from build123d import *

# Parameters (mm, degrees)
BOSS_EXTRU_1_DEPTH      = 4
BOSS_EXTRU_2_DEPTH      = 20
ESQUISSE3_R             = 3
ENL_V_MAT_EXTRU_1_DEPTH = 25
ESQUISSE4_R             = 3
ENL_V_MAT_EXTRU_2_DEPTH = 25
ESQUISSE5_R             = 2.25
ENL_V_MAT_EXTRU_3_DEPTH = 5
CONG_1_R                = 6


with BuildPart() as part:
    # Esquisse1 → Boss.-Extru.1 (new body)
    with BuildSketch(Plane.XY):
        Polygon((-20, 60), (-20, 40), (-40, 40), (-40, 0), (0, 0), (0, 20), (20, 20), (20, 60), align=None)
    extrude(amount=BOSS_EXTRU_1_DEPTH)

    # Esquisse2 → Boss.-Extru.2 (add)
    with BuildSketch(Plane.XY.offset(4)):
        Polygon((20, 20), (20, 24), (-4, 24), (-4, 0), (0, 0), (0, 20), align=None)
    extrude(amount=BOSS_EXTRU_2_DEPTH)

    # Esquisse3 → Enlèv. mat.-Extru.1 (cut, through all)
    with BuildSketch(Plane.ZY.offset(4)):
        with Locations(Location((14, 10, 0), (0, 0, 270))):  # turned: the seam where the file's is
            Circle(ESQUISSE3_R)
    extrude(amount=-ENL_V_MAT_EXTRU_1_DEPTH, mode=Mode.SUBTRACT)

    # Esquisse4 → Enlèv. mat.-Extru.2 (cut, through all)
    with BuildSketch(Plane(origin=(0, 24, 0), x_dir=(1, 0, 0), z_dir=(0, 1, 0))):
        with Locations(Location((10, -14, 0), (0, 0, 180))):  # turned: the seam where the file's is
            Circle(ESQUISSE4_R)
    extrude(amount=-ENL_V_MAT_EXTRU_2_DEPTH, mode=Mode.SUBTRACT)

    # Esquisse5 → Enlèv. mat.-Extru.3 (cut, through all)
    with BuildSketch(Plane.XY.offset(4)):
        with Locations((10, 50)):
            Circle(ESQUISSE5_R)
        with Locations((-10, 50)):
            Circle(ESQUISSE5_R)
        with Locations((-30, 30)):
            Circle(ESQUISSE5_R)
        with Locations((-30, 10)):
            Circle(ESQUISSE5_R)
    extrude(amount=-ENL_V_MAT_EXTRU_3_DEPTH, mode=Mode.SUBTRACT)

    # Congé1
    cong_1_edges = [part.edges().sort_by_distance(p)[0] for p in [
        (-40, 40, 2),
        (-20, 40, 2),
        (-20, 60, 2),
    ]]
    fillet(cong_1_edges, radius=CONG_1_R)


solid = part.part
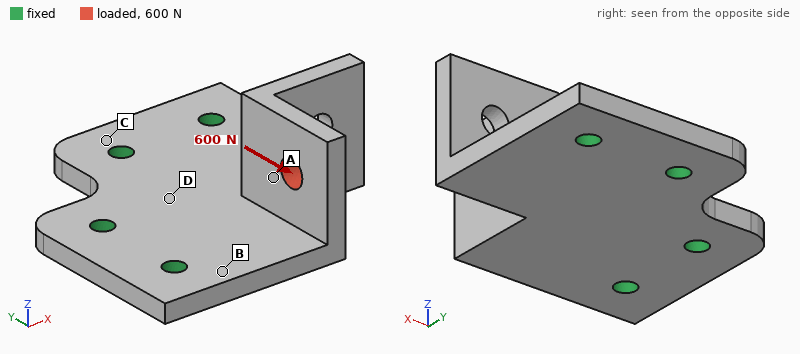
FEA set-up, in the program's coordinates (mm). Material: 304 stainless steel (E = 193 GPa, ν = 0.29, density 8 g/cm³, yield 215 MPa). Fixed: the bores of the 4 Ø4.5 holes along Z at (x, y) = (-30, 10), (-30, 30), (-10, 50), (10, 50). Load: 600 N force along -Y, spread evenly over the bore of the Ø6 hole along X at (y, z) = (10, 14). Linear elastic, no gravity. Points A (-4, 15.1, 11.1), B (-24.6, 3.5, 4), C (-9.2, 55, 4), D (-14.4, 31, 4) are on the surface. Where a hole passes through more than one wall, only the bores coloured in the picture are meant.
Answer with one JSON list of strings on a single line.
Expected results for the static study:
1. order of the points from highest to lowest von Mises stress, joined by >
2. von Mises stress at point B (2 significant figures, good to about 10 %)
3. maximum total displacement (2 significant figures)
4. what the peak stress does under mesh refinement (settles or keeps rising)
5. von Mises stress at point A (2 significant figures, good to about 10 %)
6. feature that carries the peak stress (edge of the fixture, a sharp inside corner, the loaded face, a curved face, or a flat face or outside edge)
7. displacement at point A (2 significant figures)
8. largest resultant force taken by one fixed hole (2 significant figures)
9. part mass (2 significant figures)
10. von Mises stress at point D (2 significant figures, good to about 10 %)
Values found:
["B > A > D > C", "39 MPa", "58 µm", "keeps rising", "25 MPa", "edge of the fixture", "23 µm", "290 N", "110 g", "17 MPa"]
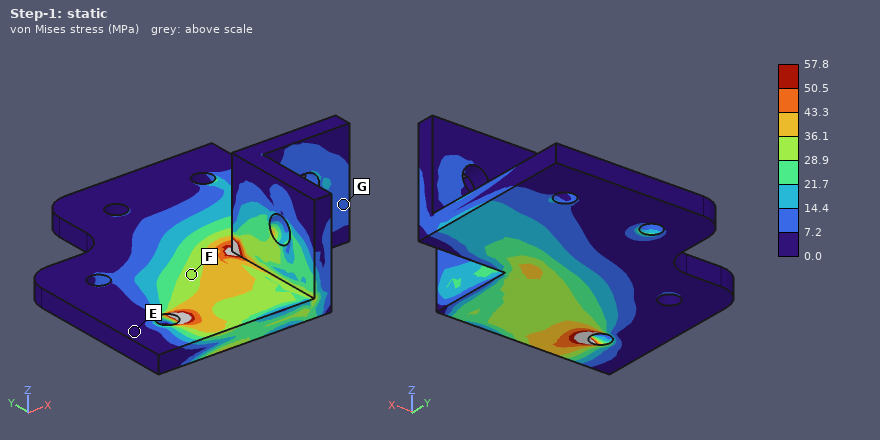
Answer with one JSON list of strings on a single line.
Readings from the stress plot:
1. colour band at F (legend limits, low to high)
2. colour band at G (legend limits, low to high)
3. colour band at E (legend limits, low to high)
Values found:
["28.9 to 36.1 MPa", "7.2 to 14.4 MPa", "0.0 to 7.2 MPa"]
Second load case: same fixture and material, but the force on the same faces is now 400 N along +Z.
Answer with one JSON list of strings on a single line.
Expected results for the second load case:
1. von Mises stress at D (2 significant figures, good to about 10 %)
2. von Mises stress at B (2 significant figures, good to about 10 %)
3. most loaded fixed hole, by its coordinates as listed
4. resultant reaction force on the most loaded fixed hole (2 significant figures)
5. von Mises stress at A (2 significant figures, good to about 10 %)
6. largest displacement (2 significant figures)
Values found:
["23 MPa", "53 MPa", "(-30, 10)", "310 N", "15 MPa", "65 µm"]
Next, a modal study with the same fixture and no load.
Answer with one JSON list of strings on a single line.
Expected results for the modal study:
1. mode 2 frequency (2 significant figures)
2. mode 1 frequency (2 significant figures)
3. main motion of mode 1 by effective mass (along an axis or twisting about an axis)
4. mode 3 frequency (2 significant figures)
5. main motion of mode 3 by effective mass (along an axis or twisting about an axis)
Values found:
["4700 Hz", "2500 Hz", "along Z", "6400 Hz", "along Z"]
